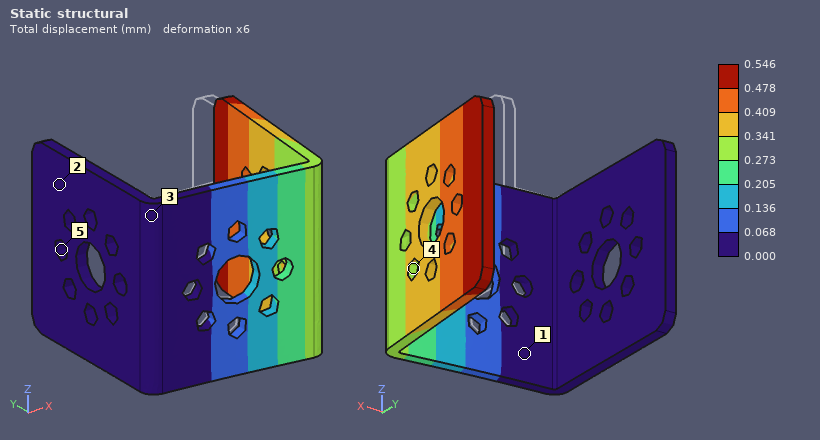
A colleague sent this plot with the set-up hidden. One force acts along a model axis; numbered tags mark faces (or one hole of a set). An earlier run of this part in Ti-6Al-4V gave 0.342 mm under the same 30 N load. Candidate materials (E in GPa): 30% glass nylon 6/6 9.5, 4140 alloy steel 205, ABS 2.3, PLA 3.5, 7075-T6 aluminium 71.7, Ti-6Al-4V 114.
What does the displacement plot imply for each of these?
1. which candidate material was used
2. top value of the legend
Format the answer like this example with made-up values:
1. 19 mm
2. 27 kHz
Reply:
1. 7075-T6 aluminium
2. 0.546 mm
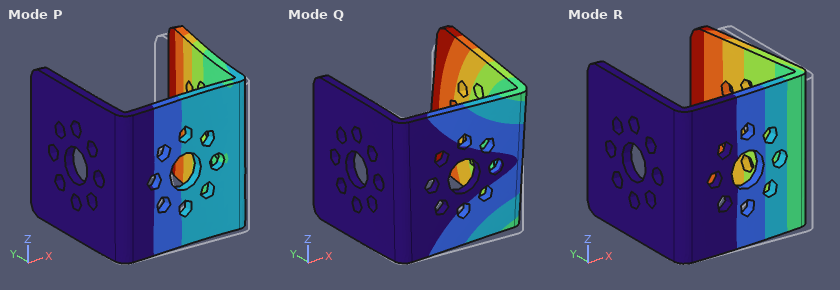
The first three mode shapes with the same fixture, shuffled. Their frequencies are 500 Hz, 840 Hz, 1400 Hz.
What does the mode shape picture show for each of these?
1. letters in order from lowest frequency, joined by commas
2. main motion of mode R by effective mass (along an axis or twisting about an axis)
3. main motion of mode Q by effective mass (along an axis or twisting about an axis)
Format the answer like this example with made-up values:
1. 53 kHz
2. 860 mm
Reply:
1. R, Q, P
2. along Y
3. along Z
